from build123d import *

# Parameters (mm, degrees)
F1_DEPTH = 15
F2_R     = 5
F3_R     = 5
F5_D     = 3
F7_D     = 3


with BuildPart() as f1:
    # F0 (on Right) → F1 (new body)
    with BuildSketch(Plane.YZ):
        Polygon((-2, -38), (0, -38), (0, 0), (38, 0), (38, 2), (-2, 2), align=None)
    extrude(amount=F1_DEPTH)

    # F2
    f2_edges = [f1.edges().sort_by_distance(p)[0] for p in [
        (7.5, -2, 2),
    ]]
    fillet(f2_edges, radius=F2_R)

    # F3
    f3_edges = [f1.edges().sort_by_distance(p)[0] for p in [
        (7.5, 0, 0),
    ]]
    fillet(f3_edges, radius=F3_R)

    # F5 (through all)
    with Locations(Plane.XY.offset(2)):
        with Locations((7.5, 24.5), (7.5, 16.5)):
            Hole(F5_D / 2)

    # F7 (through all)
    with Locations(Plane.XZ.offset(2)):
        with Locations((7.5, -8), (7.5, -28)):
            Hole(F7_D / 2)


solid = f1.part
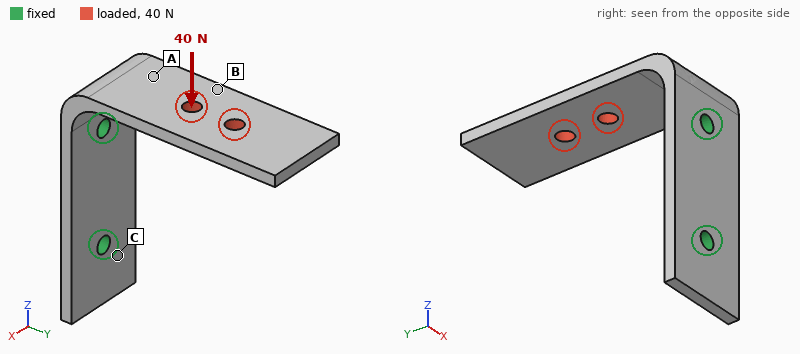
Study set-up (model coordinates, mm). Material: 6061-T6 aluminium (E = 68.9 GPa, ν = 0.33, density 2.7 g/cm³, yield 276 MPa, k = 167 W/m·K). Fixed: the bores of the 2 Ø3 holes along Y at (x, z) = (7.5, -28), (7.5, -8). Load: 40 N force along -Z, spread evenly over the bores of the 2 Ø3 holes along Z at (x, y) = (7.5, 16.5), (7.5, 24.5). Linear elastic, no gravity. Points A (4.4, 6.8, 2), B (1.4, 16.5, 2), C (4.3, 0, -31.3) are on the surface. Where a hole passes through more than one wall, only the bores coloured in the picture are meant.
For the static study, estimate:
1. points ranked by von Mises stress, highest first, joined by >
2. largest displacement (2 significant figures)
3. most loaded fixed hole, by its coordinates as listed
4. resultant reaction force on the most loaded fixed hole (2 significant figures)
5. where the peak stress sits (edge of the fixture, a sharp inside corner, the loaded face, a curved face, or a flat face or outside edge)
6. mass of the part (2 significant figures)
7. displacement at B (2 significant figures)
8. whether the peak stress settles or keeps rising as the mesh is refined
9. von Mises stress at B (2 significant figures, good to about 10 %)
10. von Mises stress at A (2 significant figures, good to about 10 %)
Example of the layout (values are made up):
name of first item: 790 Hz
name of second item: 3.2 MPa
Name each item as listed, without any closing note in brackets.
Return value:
points ranked by von Mises stress, highest first, joined by >: A > B > C
largest displacement: 0.57 mm
most loaded fixed hole, by its coordinates as listed: (7.5, -8)
resultant reaction force on the most loaded fixed hole: 39 N
where the peak stress sits: edge of the fixture
mass of the part: 6.2 g
displacement at B: 0.21 mm
whether the peak stress settles or keeps rising as the mesh is refined: keeps rising
von Mises stress at B: 21 MPa
von Mises stress at A: 50 MPa
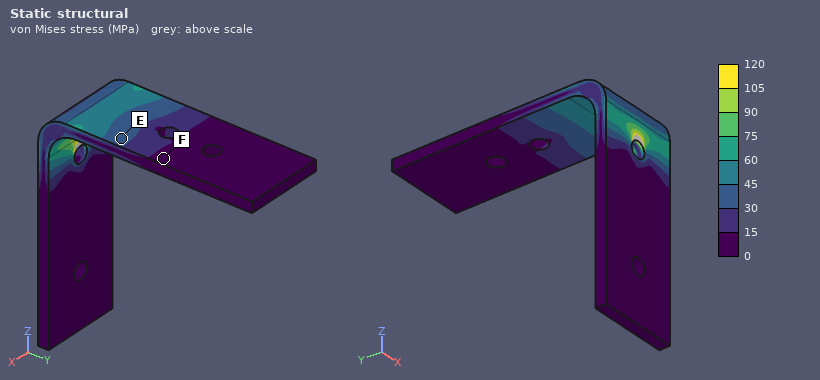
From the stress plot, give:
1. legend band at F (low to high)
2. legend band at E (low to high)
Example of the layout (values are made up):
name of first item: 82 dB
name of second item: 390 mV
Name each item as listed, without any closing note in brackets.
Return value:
legend band at F: 0 to 15 MPa
legend band at E: 30 to 45 MPa
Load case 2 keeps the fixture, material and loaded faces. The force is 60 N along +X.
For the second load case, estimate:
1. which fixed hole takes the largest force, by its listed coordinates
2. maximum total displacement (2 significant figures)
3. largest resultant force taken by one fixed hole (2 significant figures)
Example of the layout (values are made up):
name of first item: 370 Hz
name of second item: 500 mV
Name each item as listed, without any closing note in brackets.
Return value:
which fixed hole takes the largest force, by its listed coordinates: (7.5, -8)
maximum total displacement: 0.26 mm
largest resultant force taken by one fixed hole: 78 N
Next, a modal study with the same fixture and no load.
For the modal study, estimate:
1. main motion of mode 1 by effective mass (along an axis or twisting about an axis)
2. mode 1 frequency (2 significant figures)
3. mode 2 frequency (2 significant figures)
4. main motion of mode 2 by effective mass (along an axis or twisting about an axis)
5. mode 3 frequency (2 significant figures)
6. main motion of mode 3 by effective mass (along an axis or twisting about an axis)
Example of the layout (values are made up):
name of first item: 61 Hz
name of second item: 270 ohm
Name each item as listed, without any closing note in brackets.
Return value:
main motion of mode 1 by effective mass: along Z
mode 1 frequency: 950 Hz
mode 2 frequency: 1800 Hz
main motion of mode 2 by effective mass: along X
mode 3 frequency: 4800 Hz
main motion of mode 3 by effective mass: along Y
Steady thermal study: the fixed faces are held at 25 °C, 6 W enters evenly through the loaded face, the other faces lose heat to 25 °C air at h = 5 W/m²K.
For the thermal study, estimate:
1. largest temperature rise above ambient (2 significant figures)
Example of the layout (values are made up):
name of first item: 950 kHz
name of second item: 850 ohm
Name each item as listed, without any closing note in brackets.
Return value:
largest temperature rise above ambient: 34 K
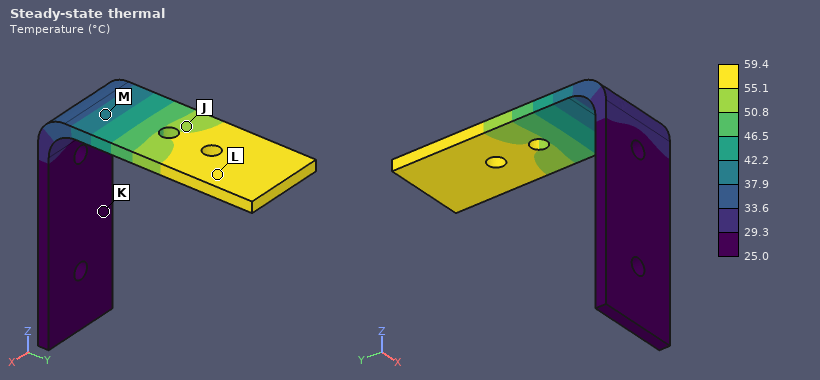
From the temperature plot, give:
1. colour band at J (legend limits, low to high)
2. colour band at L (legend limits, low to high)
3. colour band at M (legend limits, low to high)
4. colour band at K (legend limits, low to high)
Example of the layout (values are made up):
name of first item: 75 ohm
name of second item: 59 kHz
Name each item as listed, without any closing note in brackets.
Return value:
colour band at J: 50.8 to 55.1 °C
colour band at L: 55.1 to 59.4 °C
colour band at M: 37.9 to 42.2 °C
colour band at K: 25.0 to 29.3 °C
